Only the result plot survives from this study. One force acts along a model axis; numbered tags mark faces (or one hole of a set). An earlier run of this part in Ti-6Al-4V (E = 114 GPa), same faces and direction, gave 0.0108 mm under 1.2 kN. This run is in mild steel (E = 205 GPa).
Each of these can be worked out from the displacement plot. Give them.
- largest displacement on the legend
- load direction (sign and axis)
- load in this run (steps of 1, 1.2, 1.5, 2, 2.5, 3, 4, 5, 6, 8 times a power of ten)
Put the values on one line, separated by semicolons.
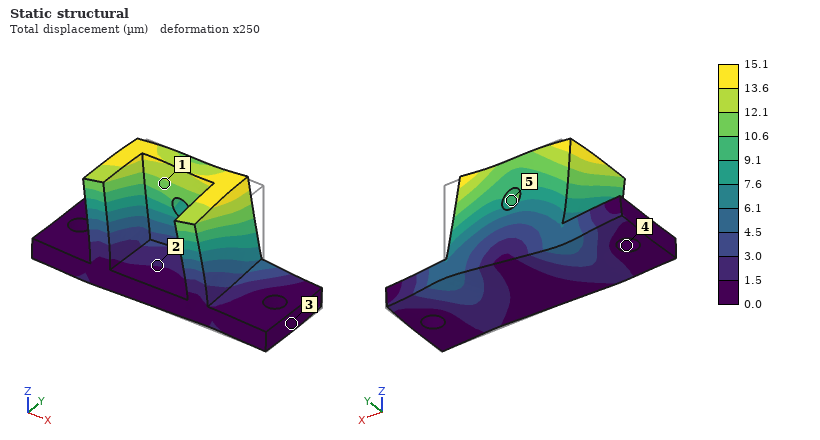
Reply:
15.1 µm; -X; 3 kN
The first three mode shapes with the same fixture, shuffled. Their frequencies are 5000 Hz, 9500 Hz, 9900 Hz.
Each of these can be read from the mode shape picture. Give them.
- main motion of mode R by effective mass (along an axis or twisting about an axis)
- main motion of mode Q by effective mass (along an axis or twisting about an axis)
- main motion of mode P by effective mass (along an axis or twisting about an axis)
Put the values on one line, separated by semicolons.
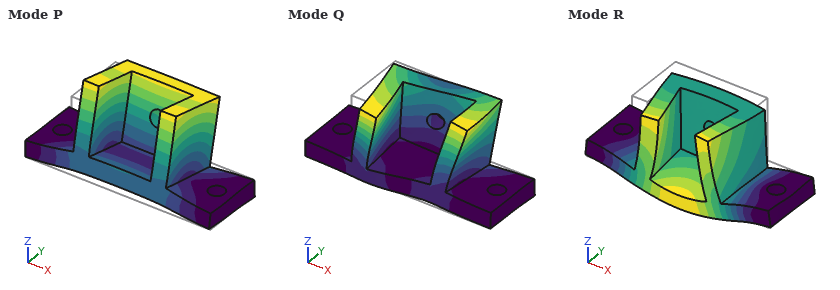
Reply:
along Z; along X; along Y
